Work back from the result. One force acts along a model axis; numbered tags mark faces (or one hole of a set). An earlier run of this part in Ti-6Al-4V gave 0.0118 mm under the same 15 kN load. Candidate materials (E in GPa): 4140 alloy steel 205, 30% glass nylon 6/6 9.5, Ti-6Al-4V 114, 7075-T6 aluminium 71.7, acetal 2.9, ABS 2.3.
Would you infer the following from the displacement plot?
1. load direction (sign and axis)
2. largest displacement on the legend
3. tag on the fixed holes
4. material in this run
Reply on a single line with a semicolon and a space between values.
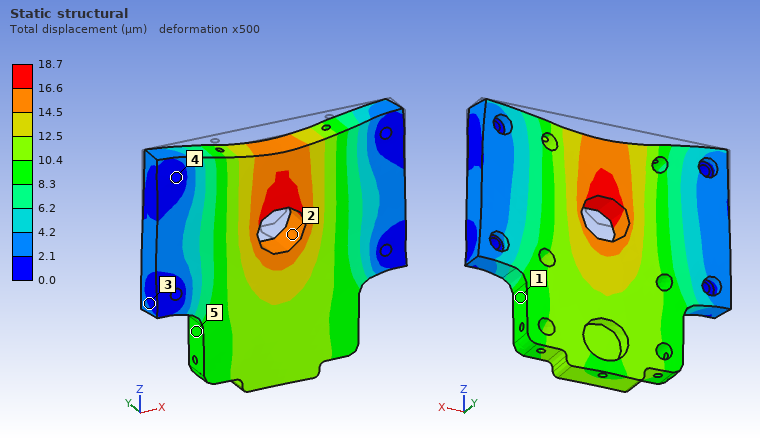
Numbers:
-Z; 18.7 µm; 4; 7075-T6 aluminium
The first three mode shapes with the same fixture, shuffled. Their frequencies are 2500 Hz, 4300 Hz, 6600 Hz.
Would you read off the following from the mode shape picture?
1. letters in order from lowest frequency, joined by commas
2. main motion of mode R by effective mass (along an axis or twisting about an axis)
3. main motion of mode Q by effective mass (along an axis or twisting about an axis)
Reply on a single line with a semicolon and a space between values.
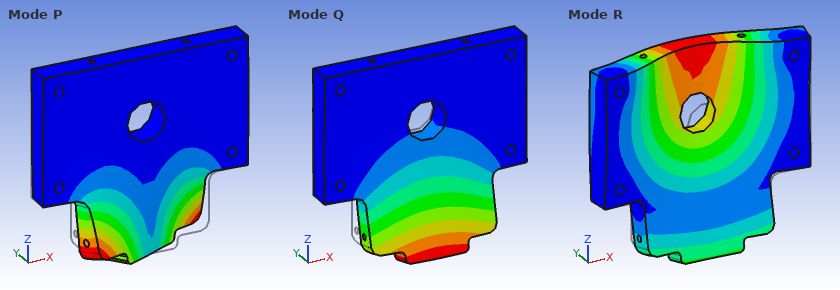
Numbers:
Q, R, P; along Y; along Y
